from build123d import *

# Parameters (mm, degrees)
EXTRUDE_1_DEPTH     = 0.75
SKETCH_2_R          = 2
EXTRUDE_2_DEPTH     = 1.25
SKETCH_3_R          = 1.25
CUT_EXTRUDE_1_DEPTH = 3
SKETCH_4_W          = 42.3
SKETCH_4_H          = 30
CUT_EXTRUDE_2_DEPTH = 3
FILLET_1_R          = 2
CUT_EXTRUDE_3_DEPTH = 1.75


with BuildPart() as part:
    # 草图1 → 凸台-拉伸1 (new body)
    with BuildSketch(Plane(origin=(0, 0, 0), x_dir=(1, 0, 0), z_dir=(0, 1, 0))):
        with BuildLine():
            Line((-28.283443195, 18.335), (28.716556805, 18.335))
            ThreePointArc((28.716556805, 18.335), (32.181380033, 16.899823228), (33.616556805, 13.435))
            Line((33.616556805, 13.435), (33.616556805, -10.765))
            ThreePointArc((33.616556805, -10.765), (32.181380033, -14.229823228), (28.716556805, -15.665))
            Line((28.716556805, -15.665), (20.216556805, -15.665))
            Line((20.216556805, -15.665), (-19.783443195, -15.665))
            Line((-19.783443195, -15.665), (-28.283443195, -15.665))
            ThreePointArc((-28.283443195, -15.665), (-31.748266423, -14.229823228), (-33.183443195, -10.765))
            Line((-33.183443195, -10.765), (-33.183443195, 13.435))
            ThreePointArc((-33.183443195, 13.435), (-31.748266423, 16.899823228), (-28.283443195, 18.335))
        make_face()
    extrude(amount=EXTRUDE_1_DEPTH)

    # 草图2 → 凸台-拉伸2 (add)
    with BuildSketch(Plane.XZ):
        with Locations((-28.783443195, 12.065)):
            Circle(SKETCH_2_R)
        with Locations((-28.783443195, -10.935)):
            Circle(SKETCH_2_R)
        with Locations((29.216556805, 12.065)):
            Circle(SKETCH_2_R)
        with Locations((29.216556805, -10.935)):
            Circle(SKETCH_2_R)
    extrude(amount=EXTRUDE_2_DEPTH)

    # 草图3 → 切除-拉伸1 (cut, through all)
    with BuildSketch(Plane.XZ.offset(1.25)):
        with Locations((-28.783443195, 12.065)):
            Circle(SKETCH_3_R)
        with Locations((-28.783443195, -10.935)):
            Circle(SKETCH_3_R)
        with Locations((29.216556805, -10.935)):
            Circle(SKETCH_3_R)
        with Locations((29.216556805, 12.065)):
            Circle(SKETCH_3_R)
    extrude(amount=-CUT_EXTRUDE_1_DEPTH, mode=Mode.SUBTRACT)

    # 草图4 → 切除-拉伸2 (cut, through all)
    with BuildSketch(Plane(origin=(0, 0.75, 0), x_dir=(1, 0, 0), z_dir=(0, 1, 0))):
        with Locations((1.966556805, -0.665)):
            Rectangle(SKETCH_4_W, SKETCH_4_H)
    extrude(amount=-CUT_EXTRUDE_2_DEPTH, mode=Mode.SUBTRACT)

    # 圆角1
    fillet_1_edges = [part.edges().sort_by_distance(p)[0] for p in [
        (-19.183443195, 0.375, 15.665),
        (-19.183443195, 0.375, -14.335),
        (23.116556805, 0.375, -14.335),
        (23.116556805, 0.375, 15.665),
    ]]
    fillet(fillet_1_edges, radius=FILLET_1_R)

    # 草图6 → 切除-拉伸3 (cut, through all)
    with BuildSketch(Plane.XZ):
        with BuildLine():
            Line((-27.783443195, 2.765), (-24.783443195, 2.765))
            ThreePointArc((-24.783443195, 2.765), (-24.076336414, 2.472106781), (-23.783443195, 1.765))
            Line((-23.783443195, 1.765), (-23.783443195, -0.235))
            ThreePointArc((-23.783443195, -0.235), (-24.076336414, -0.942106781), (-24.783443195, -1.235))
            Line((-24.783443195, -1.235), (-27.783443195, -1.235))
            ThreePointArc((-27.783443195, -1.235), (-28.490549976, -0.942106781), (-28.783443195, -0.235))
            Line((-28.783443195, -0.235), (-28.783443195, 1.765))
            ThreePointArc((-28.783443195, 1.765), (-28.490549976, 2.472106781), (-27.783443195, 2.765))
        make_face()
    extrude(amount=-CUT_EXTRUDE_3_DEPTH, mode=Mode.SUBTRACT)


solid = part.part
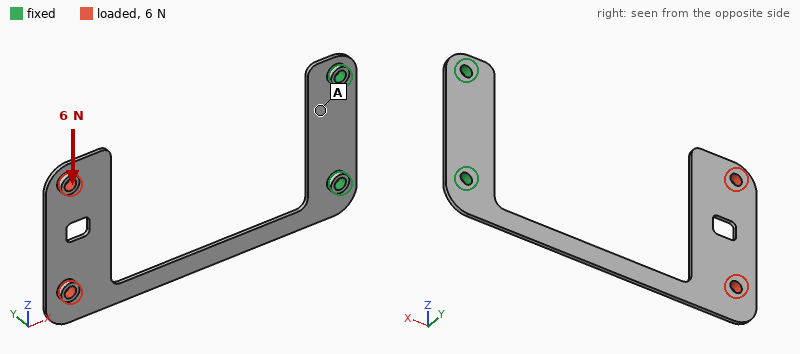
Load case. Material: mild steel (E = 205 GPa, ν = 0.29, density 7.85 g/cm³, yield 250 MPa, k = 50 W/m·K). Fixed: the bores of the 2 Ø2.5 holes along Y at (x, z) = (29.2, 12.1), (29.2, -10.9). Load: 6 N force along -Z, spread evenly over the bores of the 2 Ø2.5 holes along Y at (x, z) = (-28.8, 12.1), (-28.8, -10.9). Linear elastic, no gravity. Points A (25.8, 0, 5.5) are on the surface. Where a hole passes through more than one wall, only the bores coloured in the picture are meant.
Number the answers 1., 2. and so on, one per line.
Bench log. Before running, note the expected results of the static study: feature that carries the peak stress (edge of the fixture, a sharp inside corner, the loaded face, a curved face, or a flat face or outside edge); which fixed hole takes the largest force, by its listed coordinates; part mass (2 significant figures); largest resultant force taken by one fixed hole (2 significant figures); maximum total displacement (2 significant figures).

1. a curved face
2. (29.2, 12.1)
3. 5.9 g
4. 12 N
5. 0.53 mm
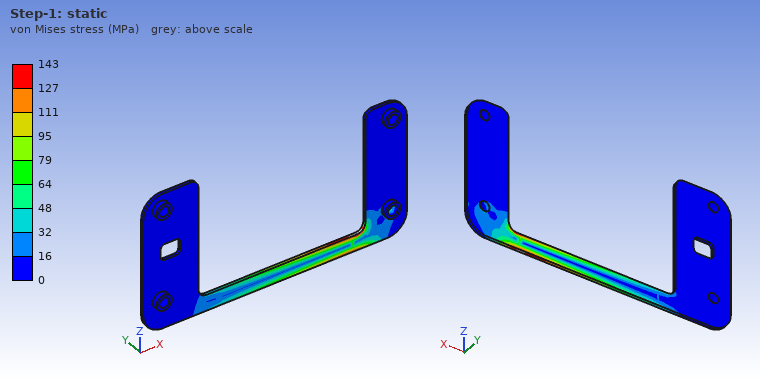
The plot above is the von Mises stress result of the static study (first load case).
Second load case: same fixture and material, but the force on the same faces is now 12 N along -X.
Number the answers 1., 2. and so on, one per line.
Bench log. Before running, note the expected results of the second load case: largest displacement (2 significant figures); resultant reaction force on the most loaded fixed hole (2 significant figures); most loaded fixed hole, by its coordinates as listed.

1. 0.67 mm
2. 9.1 N
3. (29.2, -10.9)
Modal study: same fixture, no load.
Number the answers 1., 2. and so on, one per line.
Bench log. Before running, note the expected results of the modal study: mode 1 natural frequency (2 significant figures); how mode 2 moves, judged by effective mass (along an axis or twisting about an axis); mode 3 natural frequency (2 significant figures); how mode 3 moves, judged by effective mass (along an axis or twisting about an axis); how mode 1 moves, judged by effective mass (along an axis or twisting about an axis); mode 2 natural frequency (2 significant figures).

1. 68 Hz
2. twisting about X
3. 360 Hz
4. along Z
5. along Y
6. 270 Hz
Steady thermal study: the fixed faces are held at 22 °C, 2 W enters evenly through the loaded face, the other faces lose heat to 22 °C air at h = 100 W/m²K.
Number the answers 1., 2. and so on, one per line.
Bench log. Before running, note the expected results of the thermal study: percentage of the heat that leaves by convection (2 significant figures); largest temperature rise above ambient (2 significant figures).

1. 100 %
2. 30 K
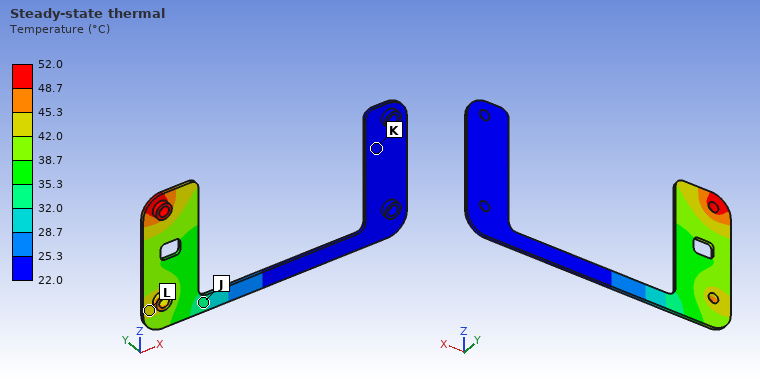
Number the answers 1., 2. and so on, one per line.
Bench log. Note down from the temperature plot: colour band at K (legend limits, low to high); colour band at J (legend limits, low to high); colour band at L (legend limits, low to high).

1. 22.0 to 25.3 °C
2. 32.0 to 35.3 °C
3. 42.0 to 45.3 °C
